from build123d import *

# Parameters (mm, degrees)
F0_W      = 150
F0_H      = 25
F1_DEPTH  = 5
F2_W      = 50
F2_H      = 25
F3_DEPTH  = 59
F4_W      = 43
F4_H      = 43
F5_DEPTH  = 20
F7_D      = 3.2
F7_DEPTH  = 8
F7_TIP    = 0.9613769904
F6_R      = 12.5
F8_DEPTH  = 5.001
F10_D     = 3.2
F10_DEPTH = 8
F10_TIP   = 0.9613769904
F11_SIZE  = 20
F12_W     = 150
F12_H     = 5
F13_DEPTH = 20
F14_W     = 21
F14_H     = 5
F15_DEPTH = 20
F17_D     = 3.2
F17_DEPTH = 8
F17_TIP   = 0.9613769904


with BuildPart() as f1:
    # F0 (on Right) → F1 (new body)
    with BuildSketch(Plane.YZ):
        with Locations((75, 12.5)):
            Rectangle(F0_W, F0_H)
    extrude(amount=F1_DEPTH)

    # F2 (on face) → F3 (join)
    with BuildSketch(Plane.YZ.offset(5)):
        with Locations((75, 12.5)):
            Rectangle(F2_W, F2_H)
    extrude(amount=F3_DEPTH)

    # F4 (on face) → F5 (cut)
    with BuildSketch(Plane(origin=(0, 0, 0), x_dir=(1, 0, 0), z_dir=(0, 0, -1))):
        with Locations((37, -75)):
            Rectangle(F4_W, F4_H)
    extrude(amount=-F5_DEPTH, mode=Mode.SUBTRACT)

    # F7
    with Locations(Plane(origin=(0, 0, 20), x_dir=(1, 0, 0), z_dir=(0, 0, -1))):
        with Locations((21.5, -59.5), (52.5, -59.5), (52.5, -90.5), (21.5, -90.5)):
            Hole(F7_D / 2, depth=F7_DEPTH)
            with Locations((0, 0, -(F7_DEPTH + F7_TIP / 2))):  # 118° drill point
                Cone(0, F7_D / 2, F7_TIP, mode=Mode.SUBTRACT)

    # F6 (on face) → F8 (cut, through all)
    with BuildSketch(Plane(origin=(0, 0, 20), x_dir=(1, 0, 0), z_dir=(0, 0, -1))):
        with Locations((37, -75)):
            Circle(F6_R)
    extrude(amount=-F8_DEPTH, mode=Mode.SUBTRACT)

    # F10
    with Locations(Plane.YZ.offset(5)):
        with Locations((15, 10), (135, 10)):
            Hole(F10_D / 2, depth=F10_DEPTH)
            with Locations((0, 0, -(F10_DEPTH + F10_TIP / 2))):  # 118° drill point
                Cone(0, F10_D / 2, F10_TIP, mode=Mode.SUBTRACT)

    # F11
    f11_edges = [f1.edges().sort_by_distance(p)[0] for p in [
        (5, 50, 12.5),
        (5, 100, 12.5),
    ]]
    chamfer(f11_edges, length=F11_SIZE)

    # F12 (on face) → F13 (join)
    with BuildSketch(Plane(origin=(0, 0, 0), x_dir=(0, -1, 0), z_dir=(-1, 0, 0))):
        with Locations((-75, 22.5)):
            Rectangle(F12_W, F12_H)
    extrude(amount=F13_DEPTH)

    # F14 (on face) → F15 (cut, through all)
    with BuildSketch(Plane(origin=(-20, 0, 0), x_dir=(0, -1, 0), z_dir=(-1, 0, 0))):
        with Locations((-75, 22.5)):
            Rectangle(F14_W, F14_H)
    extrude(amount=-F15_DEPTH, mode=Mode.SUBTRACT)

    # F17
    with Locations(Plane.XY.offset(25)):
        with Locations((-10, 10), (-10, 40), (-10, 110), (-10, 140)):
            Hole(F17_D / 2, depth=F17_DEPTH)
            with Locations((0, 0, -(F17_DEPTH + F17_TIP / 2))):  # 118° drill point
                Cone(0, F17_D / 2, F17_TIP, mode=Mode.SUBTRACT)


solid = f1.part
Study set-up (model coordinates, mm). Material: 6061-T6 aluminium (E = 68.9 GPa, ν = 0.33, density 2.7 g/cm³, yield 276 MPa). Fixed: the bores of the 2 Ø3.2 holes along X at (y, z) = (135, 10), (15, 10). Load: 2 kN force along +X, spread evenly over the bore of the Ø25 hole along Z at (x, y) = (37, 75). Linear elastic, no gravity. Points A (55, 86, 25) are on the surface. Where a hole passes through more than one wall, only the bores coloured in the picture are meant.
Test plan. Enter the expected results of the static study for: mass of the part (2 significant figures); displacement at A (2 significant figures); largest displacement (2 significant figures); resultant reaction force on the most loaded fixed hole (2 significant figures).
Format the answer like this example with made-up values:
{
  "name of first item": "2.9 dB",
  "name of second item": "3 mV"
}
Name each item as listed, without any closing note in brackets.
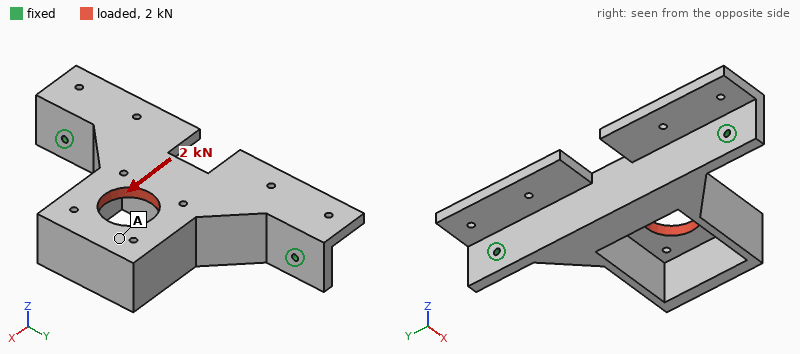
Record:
{
  "mass of the part": "200 g",
  "displacement at A": "0.31 mm",
  "largest displacement": "0.36 mm",
  "resultant reaction force on the most loaded fixed hole": "1.2 kN"
}
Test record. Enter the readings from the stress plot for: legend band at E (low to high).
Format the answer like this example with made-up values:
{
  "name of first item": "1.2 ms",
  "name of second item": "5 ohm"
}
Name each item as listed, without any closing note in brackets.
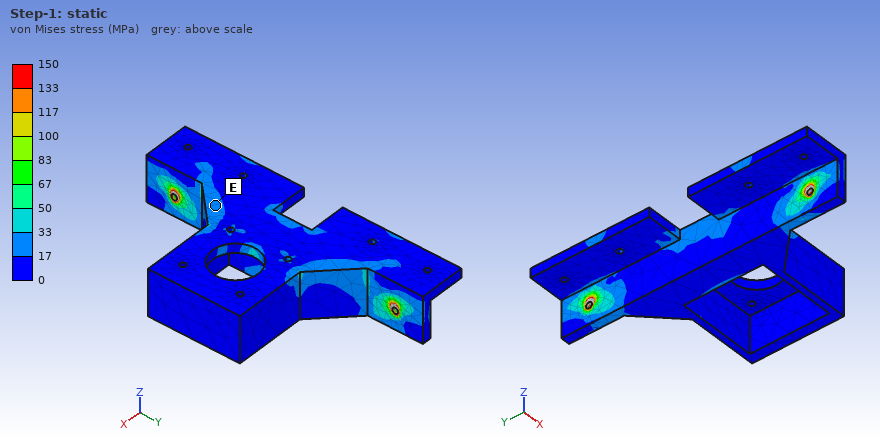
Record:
{
  "legend band at E": "17 to 33 MPa"
}
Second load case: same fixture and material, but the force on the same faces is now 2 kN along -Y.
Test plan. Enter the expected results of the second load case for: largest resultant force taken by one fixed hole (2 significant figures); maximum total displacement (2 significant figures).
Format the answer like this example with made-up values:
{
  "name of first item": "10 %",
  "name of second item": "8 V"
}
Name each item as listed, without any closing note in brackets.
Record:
{
  "largest resultant force taken by one fixed hole": "1.2 kN",
  "maximum total displacement": "58 µm"
}
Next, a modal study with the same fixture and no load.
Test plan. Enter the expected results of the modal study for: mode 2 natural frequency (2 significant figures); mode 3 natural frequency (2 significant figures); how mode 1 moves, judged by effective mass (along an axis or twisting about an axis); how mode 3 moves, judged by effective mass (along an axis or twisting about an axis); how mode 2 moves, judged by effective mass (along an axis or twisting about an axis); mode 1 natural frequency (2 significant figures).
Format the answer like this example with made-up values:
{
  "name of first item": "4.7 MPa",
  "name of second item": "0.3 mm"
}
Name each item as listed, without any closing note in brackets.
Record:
{
  "mode 2 natural frequency": "2400 Hz",
  "mode 3 natural frequency": "3000 Hz",
  "how mode 1 moves, judged by effective mass": "along Z",
  "how mode 3 moves, judged by effective mass": "along Y",
  "how mode 2 moves, judged by effective mass": "along X",
  "mode 1 natural frequency": "800 Hz"
}
